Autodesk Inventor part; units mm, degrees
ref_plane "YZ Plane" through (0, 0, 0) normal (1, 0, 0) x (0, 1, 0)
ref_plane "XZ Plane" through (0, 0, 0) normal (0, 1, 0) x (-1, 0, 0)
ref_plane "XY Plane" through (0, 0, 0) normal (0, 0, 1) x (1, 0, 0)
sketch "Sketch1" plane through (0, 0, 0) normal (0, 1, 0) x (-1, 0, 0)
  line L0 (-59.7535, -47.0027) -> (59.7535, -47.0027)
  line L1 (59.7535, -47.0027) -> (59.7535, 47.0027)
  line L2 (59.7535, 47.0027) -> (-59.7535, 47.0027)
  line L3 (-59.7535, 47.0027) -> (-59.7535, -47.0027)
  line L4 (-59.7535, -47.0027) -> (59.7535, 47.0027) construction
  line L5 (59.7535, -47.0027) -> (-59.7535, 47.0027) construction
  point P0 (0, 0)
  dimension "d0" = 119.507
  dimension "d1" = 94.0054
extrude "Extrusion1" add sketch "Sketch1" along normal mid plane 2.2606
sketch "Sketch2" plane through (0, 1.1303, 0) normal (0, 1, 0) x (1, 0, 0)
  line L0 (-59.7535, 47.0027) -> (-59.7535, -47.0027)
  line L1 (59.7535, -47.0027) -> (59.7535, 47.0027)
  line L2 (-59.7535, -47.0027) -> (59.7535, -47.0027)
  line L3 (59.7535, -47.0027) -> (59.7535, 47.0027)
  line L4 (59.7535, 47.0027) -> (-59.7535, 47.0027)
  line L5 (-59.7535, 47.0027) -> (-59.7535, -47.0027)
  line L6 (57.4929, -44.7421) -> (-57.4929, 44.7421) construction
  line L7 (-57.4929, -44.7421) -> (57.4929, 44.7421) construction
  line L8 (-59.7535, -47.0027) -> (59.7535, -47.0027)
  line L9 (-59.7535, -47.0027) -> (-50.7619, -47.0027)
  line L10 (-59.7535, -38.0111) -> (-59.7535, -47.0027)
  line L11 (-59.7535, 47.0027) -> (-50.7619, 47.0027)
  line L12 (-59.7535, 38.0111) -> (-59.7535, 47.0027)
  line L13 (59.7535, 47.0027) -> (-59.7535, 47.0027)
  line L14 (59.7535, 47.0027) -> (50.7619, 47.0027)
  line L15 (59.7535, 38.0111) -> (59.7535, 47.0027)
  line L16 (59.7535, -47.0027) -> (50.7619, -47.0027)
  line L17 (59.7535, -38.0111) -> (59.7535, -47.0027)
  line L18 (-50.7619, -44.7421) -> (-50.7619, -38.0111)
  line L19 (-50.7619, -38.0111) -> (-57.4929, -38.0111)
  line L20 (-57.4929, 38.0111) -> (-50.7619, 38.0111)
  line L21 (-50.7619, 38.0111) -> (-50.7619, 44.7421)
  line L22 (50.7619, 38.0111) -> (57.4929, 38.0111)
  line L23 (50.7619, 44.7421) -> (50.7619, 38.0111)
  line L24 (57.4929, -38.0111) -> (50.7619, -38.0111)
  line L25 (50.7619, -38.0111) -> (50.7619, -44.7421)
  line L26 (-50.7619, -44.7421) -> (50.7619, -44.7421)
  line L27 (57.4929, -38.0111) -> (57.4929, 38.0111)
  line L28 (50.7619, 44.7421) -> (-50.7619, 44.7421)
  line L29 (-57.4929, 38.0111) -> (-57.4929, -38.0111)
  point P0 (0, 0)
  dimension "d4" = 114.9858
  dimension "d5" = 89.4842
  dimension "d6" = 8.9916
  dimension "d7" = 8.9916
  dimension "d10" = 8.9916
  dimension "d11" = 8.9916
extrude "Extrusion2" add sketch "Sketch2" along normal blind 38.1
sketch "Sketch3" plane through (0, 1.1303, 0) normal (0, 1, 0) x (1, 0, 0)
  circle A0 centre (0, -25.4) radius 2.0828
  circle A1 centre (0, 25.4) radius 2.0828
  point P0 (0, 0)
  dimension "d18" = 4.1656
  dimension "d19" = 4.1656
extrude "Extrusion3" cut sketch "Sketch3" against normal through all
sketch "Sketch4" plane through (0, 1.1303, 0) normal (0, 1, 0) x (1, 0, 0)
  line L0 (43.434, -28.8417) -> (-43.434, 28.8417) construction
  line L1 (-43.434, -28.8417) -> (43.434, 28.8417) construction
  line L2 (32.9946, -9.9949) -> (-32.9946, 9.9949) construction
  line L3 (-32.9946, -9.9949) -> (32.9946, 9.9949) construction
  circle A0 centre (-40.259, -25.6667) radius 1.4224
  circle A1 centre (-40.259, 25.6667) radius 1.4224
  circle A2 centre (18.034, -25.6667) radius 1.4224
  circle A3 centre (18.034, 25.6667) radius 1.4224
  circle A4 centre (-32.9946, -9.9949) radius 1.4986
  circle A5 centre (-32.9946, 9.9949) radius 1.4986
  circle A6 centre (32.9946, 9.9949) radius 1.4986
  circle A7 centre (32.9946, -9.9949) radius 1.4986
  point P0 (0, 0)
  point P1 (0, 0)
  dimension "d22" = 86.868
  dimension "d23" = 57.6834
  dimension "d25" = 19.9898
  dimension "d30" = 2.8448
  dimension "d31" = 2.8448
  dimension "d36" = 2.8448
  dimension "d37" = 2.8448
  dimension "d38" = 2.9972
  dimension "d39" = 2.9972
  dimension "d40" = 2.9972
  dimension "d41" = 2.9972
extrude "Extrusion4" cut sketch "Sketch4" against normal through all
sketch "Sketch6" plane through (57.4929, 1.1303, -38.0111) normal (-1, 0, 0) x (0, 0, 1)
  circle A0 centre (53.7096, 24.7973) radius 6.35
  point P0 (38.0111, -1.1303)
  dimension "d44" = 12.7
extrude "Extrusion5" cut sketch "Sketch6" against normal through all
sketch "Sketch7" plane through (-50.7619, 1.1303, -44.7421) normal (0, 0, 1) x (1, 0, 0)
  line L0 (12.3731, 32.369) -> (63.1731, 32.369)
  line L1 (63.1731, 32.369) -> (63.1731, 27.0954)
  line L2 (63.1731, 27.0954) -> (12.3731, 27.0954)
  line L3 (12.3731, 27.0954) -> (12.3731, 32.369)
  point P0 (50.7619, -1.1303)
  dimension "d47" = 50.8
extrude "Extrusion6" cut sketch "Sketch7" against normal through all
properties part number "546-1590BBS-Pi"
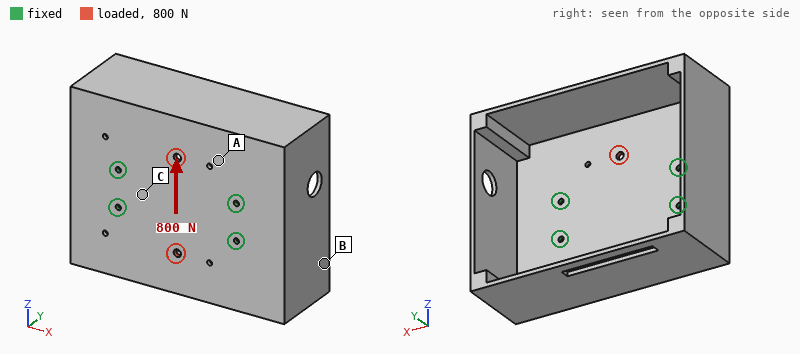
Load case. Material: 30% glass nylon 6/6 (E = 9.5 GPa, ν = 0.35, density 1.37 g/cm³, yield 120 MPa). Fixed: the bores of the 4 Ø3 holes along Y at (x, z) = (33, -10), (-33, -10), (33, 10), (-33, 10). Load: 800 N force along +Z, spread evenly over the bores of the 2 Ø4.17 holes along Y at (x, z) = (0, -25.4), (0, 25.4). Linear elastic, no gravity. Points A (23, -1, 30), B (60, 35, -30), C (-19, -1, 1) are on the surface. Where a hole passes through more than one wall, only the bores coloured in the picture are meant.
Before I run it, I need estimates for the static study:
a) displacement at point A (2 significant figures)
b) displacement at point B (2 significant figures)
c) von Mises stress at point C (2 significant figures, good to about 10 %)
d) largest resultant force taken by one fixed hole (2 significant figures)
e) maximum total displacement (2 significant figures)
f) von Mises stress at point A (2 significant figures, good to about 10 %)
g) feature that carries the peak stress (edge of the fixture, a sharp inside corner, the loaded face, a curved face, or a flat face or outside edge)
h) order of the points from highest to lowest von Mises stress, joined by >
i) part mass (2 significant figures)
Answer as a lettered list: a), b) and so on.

a) 12 µm
b) 6.5 µm
c) 4.6 MPa
d) 200 N
e) 31 µm
f) 2.6 MPa
g) the loaded face
h) C > A > B
i) 92 g
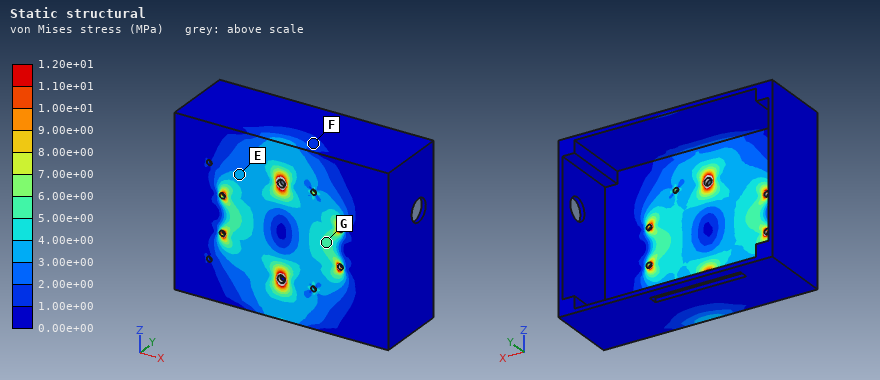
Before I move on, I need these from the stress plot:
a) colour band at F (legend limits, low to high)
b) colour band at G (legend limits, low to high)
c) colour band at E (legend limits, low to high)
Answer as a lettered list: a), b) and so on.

a) 1.00e+00 to 2.00e+00 MPa
b) 5.00e+00 to 6.00e+00 MPa
c) 3.00e+00 to 4.00e+00 MPa
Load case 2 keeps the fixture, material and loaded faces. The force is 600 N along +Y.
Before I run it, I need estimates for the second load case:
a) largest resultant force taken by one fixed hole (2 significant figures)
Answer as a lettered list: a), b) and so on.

a) 150 N
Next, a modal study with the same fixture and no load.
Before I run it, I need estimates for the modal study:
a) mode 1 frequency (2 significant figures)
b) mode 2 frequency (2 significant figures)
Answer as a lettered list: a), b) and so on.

a) 250 Hz
b) 270 Hz
